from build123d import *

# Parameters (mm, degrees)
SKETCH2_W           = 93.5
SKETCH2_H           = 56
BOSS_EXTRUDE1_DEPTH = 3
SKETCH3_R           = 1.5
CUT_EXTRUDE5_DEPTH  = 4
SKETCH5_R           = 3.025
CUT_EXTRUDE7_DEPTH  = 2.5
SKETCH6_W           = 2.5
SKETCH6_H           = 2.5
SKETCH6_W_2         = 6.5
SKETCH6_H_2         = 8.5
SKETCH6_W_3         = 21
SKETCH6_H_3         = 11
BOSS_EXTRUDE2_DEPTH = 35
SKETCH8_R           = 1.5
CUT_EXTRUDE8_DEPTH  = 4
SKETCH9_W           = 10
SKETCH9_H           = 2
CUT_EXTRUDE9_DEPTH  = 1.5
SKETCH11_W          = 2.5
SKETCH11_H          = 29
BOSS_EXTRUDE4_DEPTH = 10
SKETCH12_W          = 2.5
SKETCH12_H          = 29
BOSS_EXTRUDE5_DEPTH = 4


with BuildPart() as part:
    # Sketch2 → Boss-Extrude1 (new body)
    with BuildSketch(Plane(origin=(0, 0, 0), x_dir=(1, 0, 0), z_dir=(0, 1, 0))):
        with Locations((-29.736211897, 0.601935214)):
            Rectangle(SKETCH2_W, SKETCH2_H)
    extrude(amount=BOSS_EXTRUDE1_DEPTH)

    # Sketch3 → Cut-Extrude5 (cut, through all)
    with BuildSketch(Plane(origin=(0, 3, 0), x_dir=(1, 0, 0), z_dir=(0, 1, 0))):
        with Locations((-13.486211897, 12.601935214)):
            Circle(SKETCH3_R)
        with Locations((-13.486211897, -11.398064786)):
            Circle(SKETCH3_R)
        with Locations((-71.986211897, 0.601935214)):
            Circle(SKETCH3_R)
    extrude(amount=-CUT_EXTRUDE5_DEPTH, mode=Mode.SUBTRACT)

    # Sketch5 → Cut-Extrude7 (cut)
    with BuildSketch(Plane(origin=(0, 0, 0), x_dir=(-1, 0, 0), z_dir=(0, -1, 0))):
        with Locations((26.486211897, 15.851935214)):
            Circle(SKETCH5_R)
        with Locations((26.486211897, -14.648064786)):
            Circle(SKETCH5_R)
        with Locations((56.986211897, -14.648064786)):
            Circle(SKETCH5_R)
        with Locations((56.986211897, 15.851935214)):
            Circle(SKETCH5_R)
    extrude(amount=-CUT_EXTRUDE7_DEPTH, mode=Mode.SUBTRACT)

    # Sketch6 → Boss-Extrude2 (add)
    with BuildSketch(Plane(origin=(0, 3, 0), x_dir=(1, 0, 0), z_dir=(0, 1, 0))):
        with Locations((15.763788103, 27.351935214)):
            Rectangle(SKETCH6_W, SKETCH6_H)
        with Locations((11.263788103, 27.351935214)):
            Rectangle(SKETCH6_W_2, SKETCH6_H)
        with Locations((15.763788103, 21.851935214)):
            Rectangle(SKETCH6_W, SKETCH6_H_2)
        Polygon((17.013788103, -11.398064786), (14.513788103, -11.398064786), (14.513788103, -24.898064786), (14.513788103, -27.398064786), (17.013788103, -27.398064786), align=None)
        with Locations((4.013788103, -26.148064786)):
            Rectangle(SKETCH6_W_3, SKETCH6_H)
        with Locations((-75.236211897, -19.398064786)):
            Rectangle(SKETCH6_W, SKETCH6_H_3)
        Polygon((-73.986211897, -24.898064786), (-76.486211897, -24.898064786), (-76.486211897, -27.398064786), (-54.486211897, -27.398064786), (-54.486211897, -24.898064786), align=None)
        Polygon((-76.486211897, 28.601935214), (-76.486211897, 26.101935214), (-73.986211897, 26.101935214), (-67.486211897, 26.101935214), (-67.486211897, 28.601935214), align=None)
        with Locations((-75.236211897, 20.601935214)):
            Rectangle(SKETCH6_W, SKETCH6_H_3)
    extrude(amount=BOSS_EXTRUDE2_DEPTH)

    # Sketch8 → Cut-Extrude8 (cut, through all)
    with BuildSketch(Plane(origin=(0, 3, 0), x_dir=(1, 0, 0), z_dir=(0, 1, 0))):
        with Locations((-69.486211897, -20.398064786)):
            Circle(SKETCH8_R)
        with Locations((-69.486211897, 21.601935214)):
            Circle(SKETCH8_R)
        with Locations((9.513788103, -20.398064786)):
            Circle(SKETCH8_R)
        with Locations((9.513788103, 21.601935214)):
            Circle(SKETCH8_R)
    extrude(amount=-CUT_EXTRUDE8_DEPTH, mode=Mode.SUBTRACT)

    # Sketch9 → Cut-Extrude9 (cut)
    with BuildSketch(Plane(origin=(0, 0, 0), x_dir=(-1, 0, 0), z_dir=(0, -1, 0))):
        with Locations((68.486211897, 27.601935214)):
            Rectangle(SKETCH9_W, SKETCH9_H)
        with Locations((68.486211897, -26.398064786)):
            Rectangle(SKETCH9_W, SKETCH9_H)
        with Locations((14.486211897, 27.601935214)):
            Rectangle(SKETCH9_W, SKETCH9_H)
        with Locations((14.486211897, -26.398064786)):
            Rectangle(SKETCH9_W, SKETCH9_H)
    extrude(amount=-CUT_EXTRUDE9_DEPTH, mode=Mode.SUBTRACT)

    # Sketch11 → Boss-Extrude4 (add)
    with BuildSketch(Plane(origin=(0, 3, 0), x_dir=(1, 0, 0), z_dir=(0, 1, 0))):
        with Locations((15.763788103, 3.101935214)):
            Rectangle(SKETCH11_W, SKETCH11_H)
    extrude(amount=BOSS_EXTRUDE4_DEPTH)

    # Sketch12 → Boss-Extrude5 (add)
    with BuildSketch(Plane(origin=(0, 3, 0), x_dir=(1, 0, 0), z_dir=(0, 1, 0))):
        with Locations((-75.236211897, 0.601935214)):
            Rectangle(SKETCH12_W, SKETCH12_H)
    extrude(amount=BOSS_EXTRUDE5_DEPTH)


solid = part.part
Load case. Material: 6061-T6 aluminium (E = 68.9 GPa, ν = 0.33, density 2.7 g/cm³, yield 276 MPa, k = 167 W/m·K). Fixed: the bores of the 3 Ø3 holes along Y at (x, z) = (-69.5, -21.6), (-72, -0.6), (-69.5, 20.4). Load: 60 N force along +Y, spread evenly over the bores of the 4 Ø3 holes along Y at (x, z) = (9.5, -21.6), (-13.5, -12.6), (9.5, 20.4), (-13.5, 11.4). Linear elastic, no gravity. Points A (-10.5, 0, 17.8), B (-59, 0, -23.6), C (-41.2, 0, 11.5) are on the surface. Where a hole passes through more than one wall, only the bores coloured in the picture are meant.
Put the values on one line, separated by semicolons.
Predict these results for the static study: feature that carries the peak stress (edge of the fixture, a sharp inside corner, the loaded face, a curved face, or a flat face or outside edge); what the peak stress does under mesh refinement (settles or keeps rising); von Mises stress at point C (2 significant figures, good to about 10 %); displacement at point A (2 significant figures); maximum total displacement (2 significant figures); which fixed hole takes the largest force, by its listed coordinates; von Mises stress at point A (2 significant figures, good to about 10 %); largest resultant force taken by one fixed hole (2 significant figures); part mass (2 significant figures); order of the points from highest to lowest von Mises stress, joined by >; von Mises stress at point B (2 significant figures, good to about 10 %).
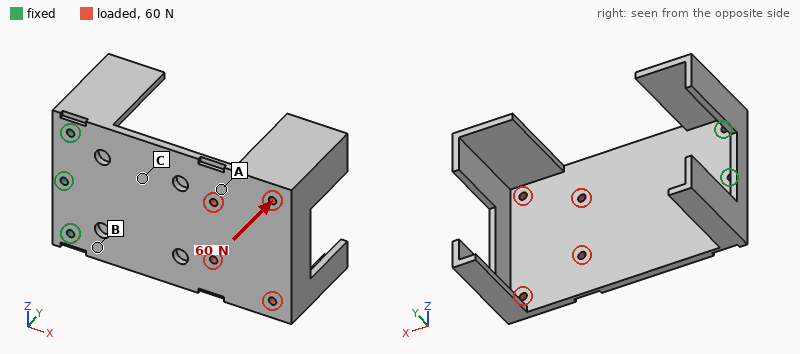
edge of the fixture; keeps rising; 28 MPa; 0.53 mm; 1.2 mm; (-72, -0.6); 9.1 MPa; 47 N; 69 g; B > C > A; 42 MPa
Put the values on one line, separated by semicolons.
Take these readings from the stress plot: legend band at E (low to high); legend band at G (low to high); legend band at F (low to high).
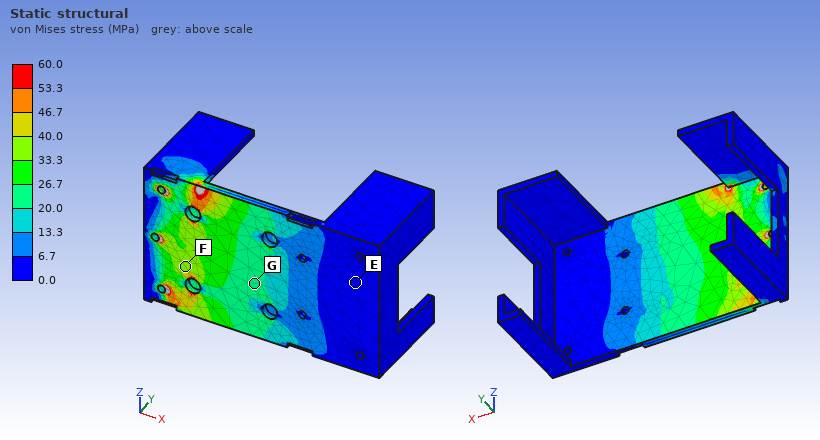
0.0 to 6.7 MPa; 20.0 to 26.7 MPa; 33.3 to 40.0 MPa
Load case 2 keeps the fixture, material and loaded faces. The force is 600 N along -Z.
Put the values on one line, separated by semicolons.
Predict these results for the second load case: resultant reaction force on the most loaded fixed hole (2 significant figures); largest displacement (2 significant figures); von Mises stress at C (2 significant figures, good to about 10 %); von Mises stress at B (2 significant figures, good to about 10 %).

980 N; 55 µm; 9.1 MPa; 22 MPa
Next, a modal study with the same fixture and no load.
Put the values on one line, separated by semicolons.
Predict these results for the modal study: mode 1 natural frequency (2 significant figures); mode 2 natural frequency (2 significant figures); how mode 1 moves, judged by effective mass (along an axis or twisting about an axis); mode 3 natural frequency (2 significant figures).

210 Hz; 550 Hz; along Y; 1100 Hz
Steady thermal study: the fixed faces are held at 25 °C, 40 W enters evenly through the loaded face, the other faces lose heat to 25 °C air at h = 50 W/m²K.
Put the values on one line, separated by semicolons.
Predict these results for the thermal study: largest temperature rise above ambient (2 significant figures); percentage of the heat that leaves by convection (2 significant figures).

50 K; 61 %
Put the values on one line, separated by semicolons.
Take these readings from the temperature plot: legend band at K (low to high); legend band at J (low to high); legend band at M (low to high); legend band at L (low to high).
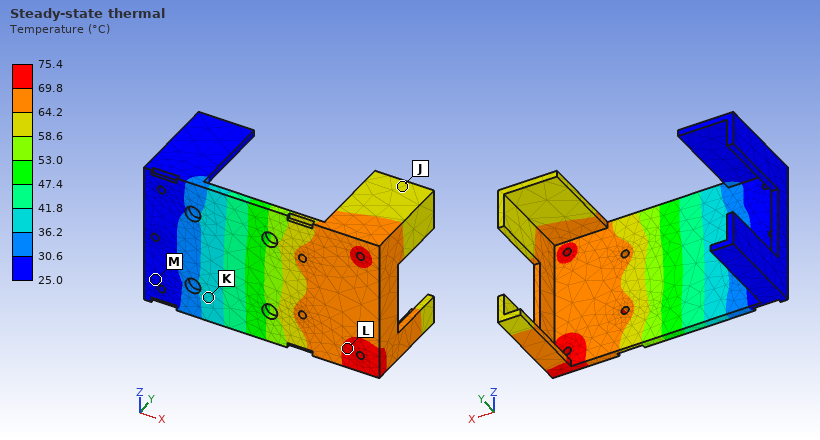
36.2 to 41.8 °C; 58.6 to 64.2 °C; 25.0 to 30.6 °C; 69.8 to 75.4 °C
